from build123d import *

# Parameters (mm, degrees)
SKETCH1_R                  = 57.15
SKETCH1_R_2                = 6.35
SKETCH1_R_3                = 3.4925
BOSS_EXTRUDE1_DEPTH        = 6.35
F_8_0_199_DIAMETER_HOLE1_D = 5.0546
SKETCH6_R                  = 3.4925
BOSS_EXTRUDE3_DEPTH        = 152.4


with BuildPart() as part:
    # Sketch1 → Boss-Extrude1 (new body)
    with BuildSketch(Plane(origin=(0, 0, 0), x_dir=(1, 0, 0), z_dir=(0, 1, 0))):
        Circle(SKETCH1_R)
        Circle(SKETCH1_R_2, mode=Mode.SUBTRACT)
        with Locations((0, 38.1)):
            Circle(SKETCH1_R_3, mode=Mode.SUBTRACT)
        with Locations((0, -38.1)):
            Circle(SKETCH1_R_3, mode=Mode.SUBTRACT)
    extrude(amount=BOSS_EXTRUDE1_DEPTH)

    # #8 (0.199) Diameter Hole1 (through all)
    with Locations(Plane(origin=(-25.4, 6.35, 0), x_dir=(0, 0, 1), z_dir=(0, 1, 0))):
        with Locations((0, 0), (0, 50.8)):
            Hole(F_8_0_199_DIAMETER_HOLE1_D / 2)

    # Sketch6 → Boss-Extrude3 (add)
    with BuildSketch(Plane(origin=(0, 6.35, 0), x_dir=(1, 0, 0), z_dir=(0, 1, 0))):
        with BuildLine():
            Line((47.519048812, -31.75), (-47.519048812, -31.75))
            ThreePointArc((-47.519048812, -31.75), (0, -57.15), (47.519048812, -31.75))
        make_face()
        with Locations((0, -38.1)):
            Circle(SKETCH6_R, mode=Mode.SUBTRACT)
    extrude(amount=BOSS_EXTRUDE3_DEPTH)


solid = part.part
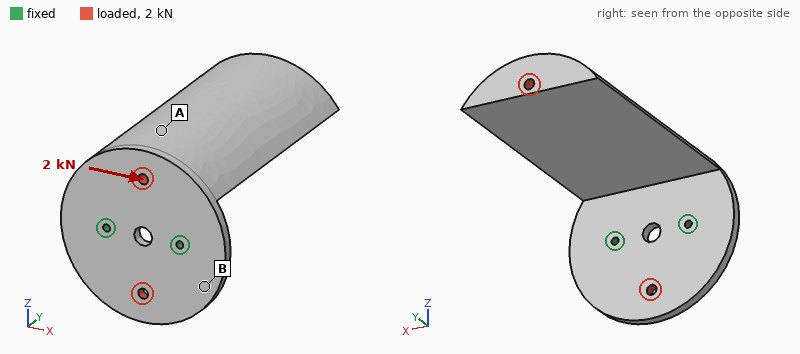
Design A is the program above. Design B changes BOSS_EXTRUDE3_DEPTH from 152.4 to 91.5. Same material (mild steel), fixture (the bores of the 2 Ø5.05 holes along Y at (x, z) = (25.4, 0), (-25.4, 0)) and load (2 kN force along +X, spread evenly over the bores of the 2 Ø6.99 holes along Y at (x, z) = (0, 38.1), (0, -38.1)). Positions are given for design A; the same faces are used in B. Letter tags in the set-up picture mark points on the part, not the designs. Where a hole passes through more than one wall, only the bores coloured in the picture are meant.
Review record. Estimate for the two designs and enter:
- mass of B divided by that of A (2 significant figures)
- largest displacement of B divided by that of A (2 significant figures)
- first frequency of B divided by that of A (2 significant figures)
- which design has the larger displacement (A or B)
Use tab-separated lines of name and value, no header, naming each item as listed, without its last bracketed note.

mass of B divided by that of A	0.68
largest displacement of B divided by that of A	0.39
first frequency of B divided by that of A	2.0
which design has the larger displacement	A
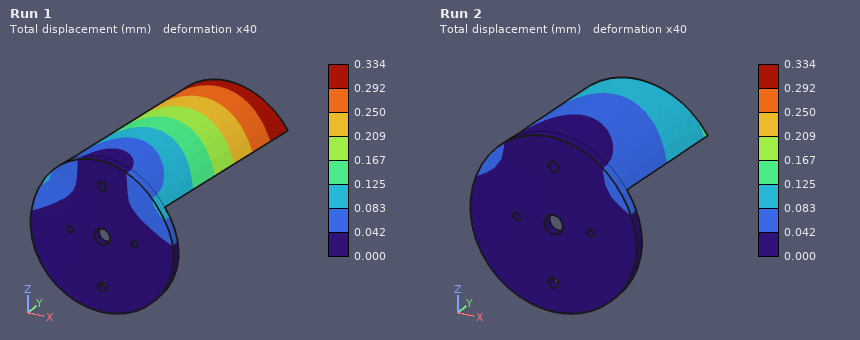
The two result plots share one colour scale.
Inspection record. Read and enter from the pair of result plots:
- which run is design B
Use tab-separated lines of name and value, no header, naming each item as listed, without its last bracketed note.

which run is design B	Run 2
